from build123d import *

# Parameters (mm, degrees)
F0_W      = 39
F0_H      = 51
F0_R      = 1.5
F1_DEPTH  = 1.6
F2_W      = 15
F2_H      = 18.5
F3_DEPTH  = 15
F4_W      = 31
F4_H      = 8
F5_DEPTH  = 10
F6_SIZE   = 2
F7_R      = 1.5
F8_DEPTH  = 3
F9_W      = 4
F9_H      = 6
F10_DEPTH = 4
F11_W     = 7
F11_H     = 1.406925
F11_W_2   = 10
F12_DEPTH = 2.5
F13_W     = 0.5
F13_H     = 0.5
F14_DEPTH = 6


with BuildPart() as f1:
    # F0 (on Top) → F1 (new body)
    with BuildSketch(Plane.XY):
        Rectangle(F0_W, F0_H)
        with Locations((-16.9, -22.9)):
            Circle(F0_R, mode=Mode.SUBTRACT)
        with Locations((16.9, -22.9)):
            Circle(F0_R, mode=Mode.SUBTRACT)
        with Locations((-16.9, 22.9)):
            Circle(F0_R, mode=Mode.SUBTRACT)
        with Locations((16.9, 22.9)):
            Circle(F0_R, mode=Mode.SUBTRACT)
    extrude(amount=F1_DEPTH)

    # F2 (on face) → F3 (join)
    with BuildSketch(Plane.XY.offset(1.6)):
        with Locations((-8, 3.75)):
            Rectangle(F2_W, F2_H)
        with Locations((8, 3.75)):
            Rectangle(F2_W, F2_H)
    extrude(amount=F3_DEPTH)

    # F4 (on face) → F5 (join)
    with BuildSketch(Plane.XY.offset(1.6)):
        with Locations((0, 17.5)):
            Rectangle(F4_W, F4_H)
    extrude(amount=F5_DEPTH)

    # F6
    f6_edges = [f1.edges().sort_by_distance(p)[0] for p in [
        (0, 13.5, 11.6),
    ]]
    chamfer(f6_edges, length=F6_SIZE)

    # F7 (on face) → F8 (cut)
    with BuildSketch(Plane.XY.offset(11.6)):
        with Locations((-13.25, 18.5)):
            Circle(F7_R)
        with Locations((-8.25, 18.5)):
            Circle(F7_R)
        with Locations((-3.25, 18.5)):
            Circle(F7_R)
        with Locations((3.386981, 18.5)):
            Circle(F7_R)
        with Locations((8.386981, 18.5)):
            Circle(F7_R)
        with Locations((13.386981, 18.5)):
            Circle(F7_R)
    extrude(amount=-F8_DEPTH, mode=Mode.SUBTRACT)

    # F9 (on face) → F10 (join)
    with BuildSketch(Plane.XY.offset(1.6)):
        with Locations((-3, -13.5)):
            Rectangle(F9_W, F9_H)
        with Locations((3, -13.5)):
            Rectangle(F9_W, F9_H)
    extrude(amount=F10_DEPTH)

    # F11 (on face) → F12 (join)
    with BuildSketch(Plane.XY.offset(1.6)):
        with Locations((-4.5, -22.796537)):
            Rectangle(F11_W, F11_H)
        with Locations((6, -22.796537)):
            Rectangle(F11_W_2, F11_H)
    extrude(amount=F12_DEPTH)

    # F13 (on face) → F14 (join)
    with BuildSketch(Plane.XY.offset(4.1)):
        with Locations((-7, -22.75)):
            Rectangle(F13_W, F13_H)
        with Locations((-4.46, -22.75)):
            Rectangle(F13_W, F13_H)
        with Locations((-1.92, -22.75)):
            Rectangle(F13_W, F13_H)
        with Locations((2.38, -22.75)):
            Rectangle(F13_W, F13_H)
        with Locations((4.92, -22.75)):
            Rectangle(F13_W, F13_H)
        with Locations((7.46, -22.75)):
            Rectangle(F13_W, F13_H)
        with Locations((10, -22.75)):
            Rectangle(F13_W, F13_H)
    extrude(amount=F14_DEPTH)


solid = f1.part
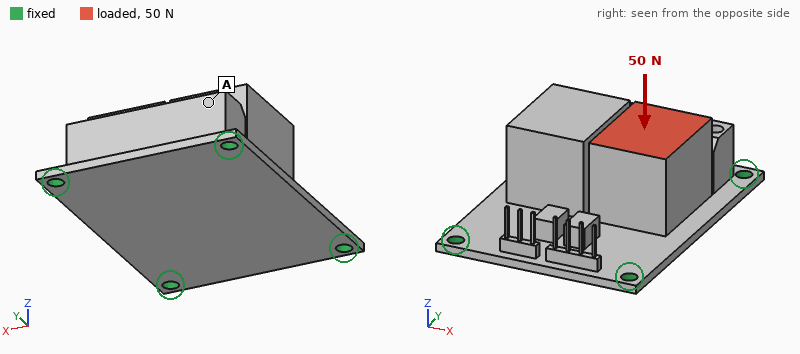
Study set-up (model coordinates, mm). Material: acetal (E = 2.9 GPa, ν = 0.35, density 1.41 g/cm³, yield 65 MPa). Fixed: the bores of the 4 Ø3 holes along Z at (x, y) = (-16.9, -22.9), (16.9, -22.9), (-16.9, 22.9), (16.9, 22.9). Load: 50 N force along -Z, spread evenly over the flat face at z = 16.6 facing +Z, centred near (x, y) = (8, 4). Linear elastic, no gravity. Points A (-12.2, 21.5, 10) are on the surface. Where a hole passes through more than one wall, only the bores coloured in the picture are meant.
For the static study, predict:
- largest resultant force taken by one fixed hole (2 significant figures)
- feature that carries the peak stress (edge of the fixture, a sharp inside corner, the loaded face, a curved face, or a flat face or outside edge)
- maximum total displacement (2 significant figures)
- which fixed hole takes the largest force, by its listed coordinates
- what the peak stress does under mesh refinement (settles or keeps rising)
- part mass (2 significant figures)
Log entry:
30 N
edge of the fixture
0.33 mm
(16.9, 22.9)
keeps rising
20 g
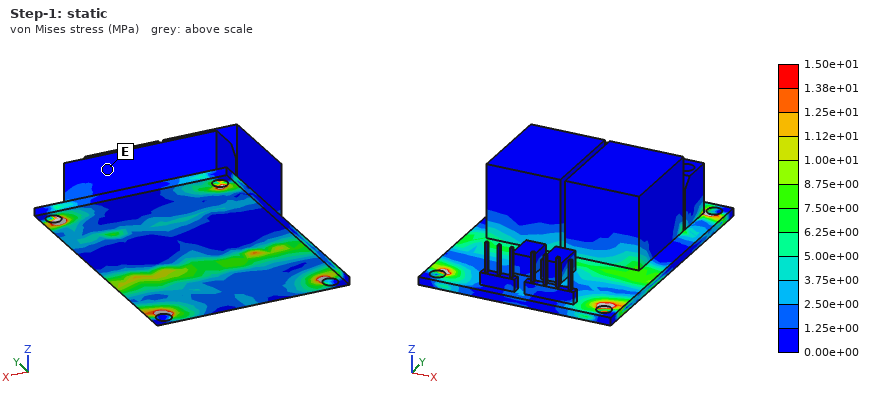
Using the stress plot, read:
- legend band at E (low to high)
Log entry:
0.00e+00 to 1.25e+00 MPa
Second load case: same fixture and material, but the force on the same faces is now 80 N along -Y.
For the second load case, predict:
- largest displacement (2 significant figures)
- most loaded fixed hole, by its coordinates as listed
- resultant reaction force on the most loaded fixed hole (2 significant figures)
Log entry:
0.52 mm
(16.9, 22.9)
37 N
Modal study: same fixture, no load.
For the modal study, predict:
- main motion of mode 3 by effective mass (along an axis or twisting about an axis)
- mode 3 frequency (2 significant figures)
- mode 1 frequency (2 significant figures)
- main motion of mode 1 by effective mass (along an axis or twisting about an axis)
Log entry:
along X
1500 Hz
580 Hz
along Z
